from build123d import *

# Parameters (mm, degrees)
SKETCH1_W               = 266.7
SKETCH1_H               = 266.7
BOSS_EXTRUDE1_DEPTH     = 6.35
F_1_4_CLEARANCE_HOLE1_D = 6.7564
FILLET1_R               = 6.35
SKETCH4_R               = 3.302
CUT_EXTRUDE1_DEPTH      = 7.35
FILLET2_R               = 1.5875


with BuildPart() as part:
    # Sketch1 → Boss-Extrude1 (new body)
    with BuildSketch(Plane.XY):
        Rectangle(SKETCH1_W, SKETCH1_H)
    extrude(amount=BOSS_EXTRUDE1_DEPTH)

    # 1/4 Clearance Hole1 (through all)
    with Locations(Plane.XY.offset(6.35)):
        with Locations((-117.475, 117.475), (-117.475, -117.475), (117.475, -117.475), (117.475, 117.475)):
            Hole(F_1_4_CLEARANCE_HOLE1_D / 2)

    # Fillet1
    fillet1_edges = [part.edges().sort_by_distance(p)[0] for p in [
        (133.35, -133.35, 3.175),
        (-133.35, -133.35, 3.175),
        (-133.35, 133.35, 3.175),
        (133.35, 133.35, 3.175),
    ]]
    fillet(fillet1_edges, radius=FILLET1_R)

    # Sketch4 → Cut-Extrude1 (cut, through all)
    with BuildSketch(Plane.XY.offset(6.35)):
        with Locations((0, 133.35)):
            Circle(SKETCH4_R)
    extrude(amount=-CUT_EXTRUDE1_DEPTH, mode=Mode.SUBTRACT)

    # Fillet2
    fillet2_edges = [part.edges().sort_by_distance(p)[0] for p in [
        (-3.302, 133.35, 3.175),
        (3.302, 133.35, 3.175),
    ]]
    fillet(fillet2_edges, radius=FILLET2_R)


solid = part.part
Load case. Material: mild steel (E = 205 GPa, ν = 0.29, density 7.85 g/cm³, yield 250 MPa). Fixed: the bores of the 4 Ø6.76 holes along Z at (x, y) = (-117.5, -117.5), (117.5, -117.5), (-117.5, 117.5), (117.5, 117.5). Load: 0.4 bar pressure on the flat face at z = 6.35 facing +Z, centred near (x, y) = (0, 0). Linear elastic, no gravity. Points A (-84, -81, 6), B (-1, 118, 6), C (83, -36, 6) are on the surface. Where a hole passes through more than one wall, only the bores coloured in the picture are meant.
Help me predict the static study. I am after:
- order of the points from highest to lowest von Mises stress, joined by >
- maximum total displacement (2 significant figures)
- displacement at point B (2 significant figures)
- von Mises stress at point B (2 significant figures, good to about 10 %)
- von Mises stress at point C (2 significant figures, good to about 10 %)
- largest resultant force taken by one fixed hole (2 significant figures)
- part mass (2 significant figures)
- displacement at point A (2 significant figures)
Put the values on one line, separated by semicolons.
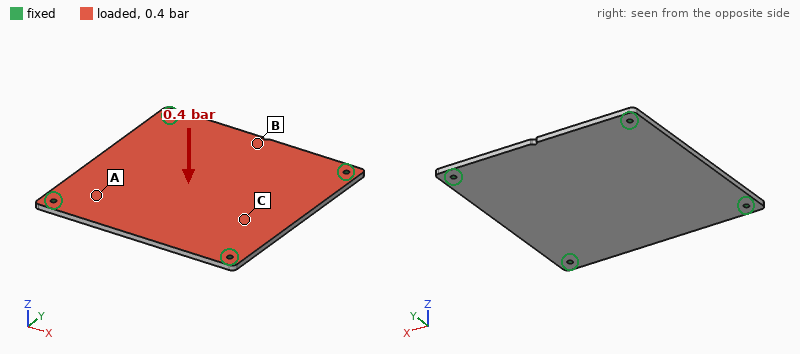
B > C > A; 0.23 mm; 0.13 mm; 22 MPa; 15 MPa; 710 N; 3.5 kg; 0.087 mm
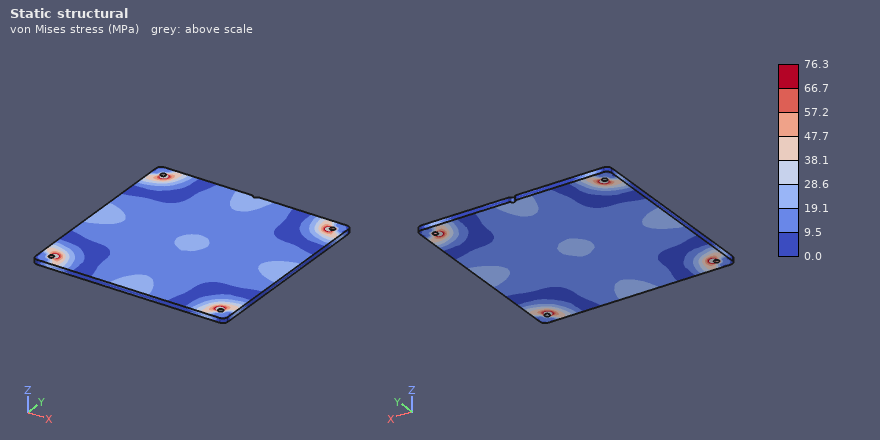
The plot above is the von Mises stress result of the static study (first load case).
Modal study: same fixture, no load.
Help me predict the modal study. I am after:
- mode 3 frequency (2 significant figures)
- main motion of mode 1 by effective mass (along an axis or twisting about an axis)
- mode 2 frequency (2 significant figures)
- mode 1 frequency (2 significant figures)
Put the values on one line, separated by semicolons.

640 Hz; along Z; 640 Hz; 360 Hz
